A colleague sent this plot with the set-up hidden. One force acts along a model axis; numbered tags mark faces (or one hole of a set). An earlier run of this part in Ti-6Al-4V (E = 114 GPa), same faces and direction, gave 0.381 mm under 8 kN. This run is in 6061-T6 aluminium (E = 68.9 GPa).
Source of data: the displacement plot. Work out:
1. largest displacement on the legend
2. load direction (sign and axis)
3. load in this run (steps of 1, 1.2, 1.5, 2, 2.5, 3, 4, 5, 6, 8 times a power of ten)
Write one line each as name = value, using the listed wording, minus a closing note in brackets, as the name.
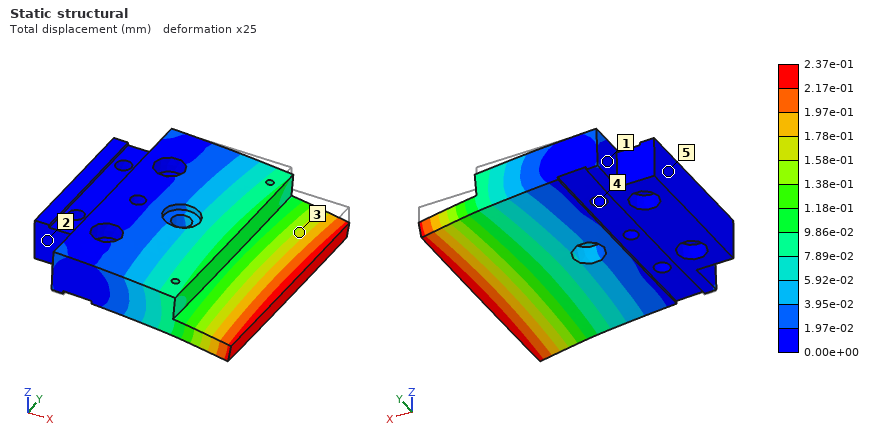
largest displacement on the legend = 2.37e-01 mm
load direction = -Z
load in this run = 3 kN
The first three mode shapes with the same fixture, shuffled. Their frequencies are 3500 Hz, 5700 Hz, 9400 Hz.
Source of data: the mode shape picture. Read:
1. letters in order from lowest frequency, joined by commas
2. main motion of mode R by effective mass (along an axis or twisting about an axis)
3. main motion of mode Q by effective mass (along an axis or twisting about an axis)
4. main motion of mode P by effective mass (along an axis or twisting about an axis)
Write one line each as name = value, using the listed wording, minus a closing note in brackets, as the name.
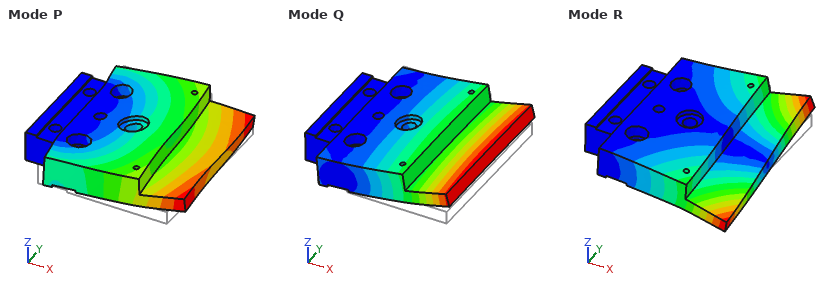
letters in order from lowest frequency, joined by commas = Q, R, P
main motion of mode R by effective mass = twisting about X
main motion of mode Q by effective mass = along Z
main motion of mode P by effective mass = along Y
